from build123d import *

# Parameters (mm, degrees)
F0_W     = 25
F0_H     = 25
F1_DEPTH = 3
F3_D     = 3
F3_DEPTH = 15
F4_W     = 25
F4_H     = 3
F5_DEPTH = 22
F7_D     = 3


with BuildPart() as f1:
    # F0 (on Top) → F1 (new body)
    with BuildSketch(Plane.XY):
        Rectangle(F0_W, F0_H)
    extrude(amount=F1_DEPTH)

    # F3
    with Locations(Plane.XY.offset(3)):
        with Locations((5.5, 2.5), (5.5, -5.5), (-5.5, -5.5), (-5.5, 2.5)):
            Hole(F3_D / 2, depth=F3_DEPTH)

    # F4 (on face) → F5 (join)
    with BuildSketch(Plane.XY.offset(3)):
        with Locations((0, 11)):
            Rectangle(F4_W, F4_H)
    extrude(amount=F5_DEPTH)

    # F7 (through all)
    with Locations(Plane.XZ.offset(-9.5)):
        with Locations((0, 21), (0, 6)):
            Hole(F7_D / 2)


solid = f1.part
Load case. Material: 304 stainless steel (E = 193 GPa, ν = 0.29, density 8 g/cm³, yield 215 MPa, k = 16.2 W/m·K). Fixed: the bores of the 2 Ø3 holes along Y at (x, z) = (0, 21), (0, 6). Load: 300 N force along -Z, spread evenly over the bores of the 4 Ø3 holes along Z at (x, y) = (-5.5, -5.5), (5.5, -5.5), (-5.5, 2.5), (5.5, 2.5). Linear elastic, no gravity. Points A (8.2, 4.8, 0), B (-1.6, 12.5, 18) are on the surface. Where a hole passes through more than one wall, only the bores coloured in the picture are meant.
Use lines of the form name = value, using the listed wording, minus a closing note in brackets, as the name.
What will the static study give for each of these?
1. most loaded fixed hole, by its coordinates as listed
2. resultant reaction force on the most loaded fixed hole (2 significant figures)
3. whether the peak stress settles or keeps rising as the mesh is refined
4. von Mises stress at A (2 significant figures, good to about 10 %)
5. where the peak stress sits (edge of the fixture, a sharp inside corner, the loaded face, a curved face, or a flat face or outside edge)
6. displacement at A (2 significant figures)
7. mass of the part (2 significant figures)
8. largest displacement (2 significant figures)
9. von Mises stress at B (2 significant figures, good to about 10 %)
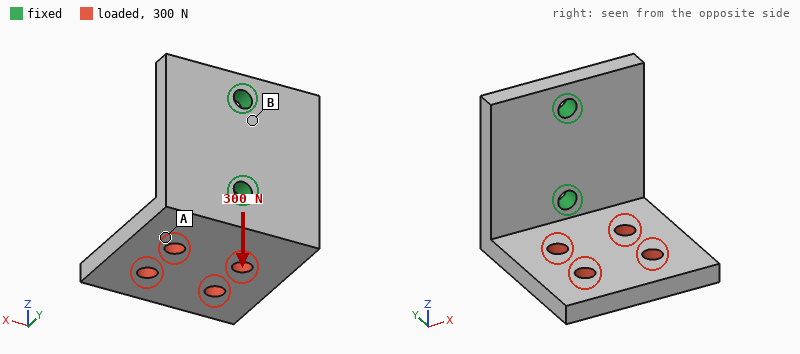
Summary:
most loaded fixed hole, by its coordinates as listed = (0, 6)
resultant reaction force on the most loaded fixed hole = 260 N
whether the peak stress settles or keeps rising as the mesh is refined = keeps rising
von Mises stress at A = 52 MPa
where the peak stress sits = edge of the fixture
displacement at A = 18 µm
mass of the part = 27 g
largest displacement = 83 µm
von Mises stress at B = 16 MPa
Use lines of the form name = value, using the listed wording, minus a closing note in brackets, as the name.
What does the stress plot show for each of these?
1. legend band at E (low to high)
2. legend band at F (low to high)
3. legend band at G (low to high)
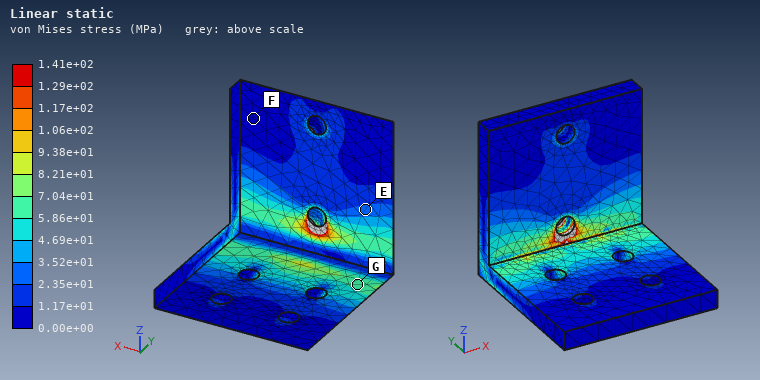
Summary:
legend band at E = 2.35e+01 to 3.52e+01 MPa
legend band at F = 0.00e+00 to 1.17e+01 MPa
legend band at G = 5.86e+01 to 7.04e+01 MPa
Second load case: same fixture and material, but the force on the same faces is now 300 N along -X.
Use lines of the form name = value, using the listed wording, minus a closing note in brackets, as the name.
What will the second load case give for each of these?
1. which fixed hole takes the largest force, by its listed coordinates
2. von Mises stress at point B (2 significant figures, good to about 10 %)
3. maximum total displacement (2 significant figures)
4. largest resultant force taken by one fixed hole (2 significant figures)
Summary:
which fixed hole takes the largest force, by its listed coordinates = (0, 6)
von Mises stress at point B = 19 MPa
maximum total displacement = 33 µm
largest resultant force taken by one fixed hole = 360 N
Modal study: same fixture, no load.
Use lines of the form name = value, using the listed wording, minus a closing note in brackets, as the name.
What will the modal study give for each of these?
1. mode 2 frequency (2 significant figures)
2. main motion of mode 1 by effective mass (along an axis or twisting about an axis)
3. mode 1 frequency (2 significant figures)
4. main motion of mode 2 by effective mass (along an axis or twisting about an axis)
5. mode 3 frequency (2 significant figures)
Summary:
mode 2 frequency = 4800 Hz
main motion of mode 1 by effective mass = along Z
mode 1 frequency = 3300 Hz
main motion of mode 2 by effective mass = along X
mode 3 frequency = 8500 Hz
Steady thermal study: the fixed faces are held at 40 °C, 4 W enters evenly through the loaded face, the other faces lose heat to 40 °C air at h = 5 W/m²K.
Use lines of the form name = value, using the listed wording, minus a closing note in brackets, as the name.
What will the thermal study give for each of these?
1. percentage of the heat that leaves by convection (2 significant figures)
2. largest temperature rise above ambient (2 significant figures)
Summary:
percentage of the heat that leaves by convection = 9.2 %
largest temperature rise above ambient = 63 K
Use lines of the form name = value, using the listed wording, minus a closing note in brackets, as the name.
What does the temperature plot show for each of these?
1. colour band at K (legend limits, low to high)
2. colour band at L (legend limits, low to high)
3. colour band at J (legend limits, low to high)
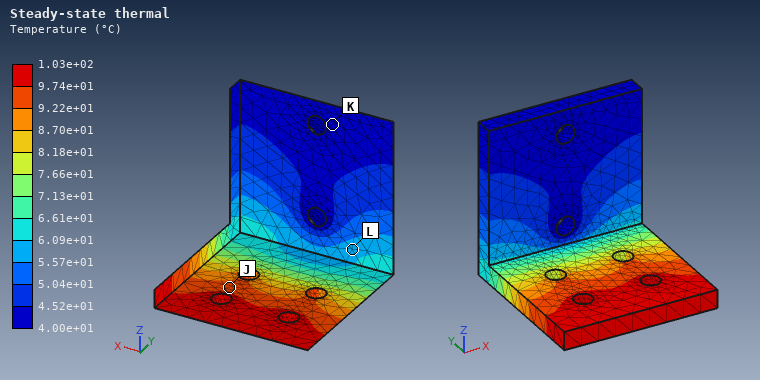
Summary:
colour band at K = 4.00e+01 to 4.52e+01 °C
colour band at L = 5.57e+01 to 6.09e+01 °C
colour band at J = 9.22e+01 to 9.74e+01 °C
